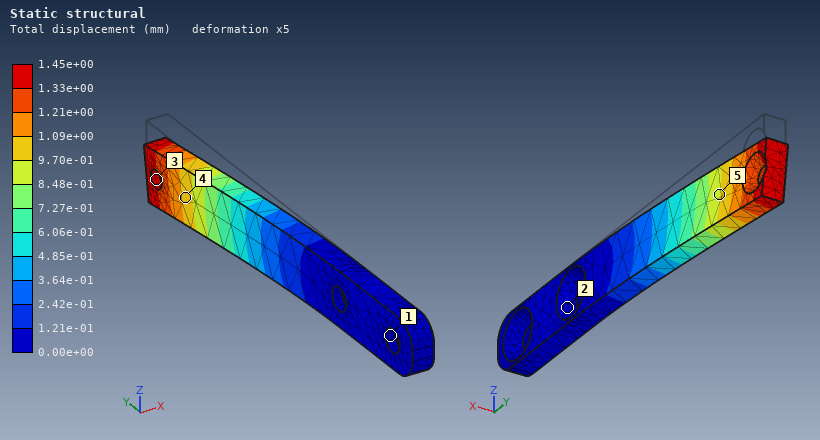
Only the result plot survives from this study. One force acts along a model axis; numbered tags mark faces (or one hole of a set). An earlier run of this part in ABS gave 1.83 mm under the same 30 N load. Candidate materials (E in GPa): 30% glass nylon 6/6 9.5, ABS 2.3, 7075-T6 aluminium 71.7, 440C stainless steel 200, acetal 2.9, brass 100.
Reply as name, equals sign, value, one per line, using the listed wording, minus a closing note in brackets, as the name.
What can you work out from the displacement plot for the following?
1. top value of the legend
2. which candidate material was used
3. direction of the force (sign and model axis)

top value of the legend = 1.45e+00 mm
which candidate material was used = acetal
direction of the force = -Z
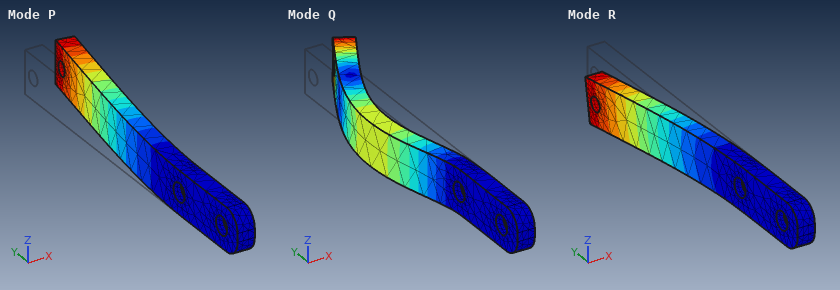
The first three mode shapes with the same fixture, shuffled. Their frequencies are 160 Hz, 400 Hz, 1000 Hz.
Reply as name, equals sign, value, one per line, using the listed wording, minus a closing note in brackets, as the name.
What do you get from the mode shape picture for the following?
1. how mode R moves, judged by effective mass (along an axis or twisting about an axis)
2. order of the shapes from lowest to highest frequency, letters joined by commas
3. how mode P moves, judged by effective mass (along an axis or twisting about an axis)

how mode R moves, judged by effective mass = along Z
order of the shapes from lowest to highest frequency, letters joined by commas = P, R, Q
how mode P moves, judged by effective mass = along X
